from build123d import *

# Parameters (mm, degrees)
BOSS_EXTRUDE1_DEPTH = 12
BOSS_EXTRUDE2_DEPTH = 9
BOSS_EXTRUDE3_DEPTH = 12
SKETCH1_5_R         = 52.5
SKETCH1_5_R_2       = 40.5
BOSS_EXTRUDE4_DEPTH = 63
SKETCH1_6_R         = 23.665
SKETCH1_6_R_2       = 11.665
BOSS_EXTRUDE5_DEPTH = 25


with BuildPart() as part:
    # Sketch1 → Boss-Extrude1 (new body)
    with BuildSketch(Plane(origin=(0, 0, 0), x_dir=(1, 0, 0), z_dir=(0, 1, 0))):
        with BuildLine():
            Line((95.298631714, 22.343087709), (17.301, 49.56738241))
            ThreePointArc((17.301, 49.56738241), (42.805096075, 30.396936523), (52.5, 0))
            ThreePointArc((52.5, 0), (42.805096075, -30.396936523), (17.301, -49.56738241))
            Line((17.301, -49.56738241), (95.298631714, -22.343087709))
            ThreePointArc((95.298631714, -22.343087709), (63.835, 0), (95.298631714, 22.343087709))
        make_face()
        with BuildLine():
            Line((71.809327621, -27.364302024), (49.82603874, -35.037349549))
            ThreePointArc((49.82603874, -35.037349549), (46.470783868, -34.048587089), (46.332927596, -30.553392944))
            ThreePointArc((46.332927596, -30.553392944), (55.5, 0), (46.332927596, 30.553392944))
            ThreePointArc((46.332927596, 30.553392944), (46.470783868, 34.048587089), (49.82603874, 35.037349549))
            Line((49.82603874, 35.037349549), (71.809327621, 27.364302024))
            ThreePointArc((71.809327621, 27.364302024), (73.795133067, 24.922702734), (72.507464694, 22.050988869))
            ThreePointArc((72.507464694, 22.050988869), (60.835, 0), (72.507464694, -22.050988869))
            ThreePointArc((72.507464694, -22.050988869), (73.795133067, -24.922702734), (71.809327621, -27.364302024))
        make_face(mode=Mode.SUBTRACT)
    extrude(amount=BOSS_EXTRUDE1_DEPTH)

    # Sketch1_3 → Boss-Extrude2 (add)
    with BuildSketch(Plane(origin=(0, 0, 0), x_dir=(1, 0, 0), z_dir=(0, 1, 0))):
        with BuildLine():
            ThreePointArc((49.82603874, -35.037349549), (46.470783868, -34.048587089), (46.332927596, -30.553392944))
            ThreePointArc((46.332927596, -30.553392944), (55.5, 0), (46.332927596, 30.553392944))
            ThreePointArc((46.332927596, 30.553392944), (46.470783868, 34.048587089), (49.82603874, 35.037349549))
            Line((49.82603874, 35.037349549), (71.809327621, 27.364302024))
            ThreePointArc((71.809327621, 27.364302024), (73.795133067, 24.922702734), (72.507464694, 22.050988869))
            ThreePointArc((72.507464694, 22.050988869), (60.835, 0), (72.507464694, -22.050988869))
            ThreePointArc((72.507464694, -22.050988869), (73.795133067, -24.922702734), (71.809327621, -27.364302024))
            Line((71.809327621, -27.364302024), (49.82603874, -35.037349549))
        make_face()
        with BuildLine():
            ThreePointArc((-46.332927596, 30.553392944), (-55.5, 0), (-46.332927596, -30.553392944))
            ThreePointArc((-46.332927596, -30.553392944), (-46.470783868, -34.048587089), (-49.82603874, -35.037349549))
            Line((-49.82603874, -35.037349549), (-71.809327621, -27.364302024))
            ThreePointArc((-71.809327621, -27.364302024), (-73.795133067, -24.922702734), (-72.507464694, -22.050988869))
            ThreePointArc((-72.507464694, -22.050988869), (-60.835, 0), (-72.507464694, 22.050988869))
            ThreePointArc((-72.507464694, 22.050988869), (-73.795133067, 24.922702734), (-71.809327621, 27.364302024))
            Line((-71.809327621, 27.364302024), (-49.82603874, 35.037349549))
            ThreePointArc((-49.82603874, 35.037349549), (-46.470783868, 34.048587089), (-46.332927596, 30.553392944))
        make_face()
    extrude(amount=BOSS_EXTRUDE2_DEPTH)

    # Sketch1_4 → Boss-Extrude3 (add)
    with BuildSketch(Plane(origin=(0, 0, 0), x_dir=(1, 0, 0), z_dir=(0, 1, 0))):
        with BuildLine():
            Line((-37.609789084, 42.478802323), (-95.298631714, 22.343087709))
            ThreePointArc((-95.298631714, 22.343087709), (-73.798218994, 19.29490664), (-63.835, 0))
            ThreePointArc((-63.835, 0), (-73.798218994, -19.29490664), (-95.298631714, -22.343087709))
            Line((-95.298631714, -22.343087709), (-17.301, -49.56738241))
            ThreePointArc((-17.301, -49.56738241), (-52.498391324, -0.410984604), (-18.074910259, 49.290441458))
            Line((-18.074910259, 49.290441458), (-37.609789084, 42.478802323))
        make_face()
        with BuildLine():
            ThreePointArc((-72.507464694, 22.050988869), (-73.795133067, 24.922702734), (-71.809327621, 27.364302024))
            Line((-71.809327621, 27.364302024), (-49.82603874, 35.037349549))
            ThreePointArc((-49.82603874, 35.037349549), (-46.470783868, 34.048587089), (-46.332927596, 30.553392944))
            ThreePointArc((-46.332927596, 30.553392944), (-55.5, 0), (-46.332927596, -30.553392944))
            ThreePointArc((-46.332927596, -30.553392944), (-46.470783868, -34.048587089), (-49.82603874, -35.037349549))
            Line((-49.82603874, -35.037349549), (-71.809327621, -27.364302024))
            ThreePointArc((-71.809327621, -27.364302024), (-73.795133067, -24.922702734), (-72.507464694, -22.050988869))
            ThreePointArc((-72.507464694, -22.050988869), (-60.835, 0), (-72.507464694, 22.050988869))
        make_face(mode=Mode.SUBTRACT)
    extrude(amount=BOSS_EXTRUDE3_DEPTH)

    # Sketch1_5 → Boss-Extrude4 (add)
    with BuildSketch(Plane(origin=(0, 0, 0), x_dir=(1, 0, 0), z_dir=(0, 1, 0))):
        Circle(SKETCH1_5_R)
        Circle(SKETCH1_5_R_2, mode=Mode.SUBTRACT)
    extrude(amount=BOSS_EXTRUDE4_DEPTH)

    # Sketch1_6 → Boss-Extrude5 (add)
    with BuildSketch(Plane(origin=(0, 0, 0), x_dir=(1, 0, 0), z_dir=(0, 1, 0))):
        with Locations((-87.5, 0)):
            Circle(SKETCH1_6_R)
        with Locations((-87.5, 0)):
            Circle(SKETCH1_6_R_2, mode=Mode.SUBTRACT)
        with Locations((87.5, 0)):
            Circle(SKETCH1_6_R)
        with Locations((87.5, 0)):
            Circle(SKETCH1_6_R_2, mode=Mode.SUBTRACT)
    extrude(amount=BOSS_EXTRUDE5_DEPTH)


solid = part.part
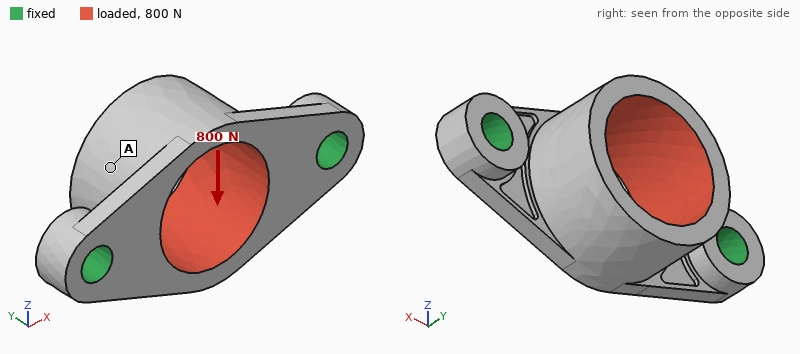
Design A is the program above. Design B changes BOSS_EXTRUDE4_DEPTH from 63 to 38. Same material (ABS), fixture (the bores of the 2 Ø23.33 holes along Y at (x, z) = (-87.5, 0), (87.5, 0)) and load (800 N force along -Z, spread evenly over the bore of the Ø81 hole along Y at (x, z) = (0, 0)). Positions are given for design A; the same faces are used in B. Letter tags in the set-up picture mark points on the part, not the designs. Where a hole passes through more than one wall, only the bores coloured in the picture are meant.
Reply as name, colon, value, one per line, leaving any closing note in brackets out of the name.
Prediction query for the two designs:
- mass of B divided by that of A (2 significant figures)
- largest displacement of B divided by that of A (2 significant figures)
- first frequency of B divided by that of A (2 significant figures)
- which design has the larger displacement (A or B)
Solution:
mass of B divided by that of A: 0.73
largest displacement of B divided by that of A: 0.47
first frequency of B divided by that of A: 1.5
which design has the larger displacement: A
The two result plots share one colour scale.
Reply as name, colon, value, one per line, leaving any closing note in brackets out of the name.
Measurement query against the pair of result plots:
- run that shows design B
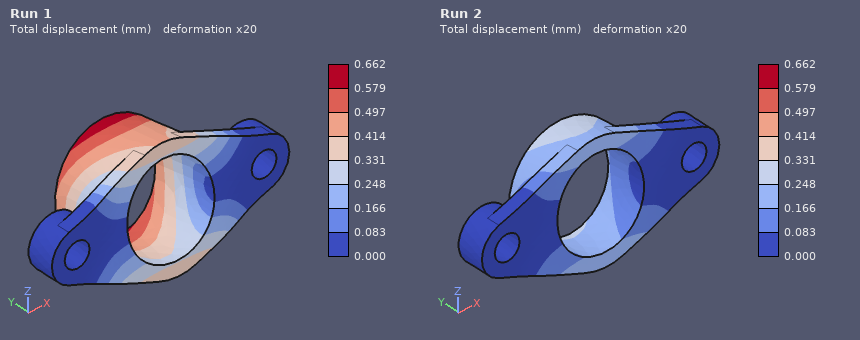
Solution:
run that shows design B: Run 2
